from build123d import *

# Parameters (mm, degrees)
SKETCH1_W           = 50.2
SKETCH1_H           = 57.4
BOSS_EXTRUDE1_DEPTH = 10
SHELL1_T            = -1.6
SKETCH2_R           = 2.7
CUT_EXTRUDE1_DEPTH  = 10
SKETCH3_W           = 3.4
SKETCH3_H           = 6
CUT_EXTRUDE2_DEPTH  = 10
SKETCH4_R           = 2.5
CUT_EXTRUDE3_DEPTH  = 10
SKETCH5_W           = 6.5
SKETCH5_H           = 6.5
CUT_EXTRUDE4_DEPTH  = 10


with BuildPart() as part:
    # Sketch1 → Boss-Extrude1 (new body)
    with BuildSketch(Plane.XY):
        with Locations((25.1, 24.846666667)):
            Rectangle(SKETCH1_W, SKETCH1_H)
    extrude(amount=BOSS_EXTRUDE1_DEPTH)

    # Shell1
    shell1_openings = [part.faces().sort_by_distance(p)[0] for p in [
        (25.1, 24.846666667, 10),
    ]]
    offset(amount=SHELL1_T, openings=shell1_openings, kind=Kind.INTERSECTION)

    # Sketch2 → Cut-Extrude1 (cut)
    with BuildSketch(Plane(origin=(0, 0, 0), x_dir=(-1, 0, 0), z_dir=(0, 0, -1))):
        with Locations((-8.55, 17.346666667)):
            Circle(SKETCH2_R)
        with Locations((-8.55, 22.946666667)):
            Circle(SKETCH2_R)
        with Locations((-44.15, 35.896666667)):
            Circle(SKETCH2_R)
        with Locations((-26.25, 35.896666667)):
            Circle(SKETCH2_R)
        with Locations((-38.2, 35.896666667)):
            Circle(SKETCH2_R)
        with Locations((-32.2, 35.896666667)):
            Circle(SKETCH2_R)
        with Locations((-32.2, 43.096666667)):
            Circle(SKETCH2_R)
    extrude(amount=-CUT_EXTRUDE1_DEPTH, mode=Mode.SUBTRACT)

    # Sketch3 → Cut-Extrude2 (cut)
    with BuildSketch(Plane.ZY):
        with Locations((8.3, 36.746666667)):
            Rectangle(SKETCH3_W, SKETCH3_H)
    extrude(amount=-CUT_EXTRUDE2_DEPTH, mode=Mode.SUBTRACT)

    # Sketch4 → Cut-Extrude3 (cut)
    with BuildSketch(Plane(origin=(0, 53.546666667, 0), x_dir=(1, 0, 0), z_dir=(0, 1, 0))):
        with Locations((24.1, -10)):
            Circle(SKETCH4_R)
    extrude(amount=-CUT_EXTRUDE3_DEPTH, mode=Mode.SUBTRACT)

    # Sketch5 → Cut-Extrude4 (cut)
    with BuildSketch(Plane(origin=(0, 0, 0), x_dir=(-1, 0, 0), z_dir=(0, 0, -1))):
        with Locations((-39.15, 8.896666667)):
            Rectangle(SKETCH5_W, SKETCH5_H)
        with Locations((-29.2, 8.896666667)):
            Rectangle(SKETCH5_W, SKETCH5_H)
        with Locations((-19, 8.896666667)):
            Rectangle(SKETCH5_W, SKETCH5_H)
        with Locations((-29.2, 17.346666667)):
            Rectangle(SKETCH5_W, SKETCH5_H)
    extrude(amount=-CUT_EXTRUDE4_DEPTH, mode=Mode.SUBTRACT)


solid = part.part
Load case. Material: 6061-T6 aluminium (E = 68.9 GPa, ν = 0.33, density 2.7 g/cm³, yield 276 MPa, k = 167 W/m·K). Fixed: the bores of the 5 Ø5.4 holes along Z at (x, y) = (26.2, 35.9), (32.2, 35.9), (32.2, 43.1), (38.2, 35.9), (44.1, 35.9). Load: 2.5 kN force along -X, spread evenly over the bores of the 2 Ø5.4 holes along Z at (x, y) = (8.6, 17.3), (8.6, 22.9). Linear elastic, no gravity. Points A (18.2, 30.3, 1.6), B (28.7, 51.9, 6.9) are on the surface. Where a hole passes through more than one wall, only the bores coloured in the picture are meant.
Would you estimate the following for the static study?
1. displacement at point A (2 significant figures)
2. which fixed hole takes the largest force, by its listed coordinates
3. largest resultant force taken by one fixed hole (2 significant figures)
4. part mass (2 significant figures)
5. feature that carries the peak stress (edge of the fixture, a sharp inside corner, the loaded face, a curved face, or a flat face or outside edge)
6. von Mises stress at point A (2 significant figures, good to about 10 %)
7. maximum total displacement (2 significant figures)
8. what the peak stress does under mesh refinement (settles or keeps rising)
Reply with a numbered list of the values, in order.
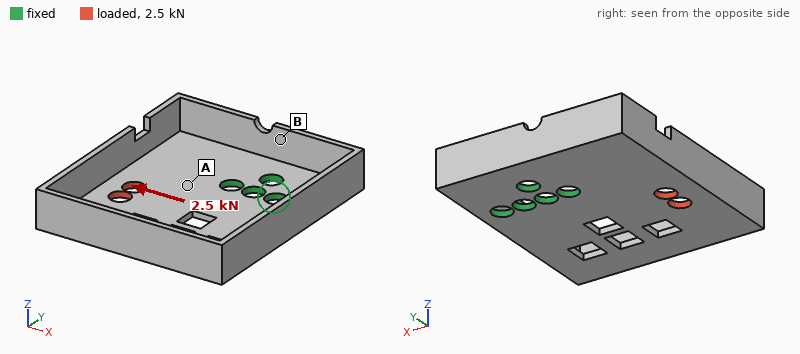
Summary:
1. 0.026 mm
2. (26.2, 35.9)
3. 2.2 kN
4. 18 g
5. a sharp inside corner
6. 78 MPa
7. 0.12 mm
8. keeps rising
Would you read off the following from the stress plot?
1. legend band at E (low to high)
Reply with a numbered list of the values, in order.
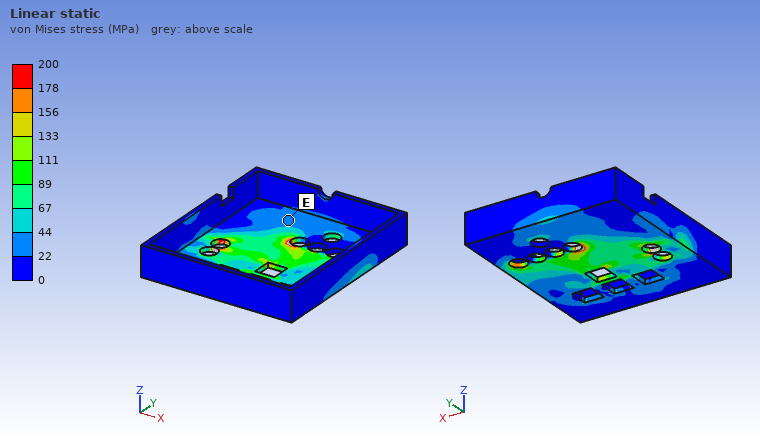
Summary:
1. 22 to 44 MPa
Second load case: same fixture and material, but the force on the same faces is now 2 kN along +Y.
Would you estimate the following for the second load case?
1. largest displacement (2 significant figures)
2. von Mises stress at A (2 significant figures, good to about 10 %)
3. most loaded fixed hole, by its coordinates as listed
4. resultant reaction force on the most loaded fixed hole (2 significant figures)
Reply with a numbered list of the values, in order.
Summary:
1. 0.11 mm
2. 83 MPa
3. (26.2, 35.9)
4. 2.6 kN
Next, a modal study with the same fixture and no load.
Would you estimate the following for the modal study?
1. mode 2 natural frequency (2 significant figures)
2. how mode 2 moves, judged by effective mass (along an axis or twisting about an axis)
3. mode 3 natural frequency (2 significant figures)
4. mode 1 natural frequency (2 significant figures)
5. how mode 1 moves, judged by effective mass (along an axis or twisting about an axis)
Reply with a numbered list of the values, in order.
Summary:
1. 2000 Hz
2. along Z
3. 2400 Hz
4. 830 Hz
5. along Z
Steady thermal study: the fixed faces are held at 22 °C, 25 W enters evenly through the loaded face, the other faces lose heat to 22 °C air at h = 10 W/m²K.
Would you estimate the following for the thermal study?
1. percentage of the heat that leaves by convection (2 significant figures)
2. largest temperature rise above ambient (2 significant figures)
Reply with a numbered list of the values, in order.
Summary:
1. 8.6 %
2. 83 K
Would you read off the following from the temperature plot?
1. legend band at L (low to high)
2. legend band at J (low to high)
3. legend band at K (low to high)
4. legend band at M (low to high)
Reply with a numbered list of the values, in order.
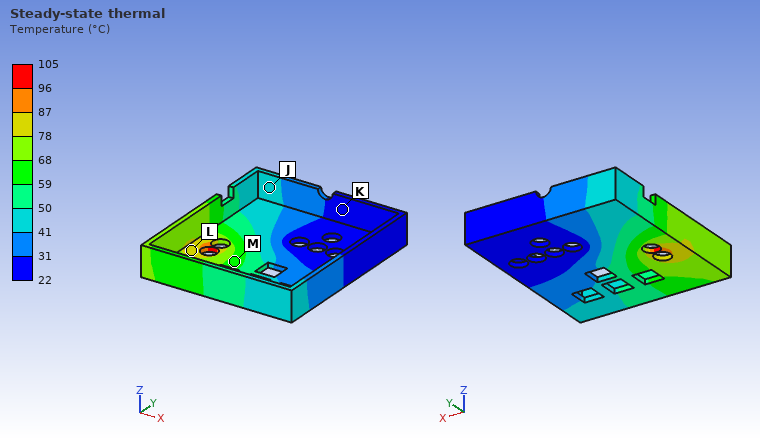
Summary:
1. 78 to 87 °C
2. 41 to 50 °C
3. 22 to 31 °C
4. 59 to 68 °C
